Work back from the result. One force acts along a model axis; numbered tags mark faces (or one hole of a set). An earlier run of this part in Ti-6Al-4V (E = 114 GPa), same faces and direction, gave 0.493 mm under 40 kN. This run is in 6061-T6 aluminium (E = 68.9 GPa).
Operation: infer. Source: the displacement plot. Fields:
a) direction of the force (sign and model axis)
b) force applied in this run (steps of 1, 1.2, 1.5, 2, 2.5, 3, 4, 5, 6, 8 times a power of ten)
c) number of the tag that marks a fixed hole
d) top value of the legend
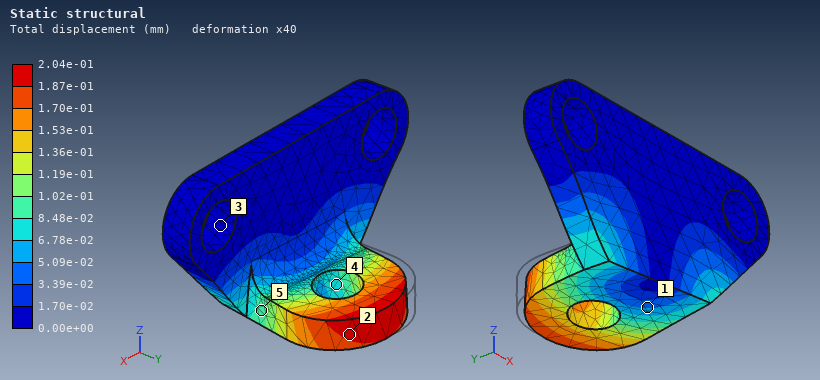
+X
10 kN
3
2.04e-01 mm
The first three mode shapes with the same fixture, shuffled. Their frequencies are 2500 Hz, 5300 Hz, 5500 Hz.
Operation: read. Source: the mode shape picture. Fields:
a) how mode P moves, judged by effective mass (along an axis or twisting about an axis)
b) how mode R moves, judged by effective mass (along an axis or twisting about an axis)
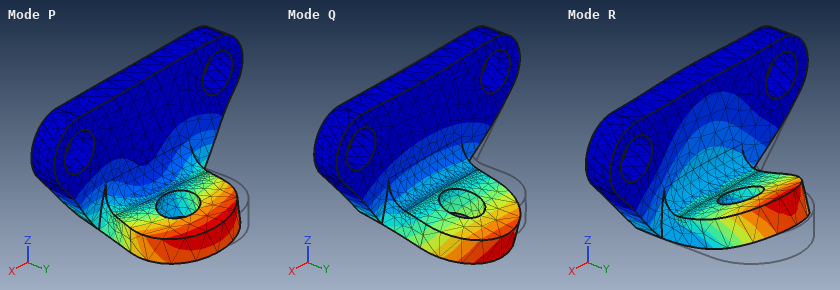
along X
along Y
